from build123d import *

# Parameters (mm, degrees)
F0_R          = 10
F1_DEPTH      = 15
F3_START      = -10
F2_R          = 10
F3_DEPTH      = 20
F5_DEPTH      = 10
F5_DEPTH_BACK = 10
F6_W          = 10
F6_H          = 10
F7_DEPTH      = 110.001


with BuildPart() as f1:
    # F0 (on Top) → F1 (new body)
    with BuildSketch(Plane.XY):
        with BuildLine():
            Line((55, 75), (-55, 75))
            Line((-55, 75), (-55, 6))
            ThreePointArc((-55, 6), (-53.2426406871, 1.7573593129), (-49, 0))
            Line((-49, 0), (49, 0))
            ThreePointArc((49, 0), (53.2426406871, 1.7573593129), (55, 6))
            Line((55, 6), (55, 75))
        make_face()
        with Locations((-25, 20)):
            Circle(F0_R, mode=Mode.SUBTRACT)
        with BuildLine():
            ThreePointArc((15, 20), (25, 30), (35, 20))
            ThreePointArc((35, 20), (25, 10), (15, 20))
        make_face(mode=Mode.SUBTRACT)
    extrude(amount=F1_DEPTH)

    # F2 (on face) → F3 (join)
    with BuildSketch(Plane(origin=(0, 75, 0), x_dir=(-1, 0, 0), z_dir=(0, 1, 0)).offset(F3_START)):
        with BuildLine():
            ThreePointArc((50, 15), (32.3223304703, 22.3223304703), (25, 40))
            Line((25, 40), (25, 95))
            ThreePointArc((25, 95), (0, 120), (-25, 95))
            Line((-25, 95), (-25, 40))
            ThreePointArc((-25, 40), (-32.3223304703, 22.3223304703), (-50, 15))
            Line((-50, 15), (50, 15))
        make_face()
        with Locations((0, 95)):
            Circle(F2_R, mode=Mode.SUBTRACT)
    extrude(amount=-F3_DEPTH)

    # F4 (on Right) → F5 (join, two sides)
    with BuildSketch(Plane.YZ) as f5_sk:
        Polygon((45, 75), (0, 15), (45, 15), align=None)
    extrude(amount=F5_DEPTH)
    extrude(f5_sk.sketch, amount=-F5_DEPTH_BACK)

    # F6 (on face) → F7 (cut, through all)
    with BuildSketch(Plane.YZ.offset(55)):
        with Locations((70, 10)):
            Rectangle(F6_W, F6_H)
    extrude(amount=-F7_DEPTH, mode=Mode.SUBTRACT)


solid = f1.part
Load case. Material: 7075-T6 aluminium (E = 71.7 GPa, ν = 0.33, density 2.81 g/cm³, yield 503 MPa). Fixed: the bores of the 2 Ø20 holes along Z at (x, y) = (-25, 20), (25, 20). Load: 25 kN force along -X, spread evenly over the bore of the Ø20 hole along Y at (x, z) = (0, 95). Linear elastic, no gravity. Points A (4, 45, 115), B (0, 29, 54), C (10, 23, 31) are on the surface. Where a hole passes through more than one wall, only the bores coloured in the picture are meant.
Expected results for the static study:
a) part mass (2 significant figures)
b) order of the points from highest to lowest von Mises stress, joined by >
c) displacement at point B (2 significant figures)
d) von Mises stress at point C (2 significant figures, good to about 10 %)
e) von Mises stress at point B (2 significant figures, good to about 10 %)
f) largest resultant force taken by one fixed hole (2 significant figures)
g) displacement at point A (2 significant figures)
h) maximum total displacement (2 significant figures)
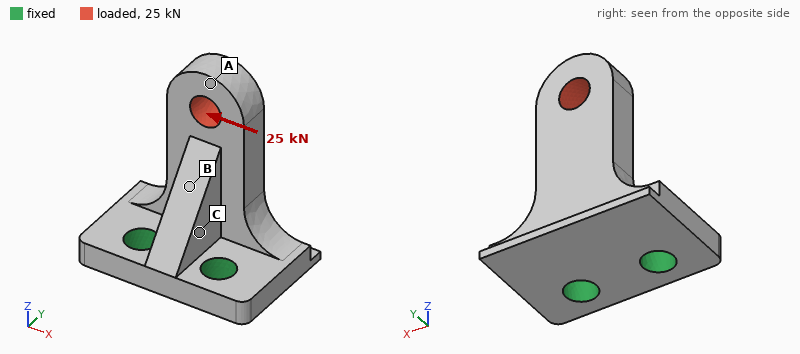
640 g
C > B > A
0.25 mm
110 MPa
73 MPa
46 kN
0.85 mm
0.90 mm
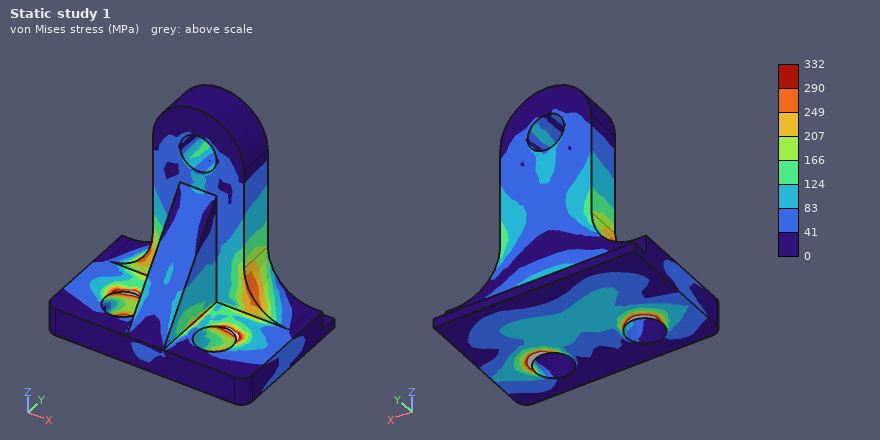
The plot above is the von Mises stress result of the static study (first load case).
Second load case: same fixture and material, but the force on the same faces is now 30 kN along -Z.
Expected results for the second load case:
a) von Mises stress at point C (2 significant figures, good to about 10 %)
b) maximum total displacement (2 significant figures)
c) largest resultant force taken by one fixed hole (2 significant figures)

28 MPa
0.41 mm
15 kN
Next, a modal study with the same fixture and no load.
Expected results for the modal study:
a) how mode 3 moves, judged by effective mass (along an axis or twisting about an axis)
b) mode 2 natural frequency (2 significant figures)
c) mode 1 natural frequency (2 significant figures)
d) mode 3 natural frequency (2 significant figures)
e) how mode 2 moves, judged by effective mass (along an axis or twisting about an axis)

along Z
2600 Hz
2000 Hz
5600 Hz
along X
